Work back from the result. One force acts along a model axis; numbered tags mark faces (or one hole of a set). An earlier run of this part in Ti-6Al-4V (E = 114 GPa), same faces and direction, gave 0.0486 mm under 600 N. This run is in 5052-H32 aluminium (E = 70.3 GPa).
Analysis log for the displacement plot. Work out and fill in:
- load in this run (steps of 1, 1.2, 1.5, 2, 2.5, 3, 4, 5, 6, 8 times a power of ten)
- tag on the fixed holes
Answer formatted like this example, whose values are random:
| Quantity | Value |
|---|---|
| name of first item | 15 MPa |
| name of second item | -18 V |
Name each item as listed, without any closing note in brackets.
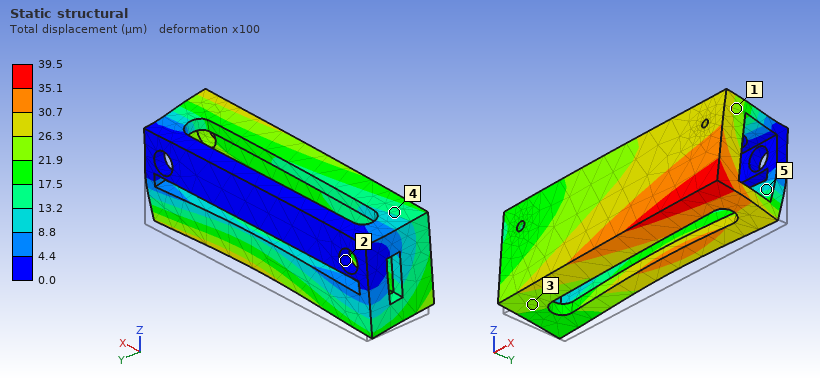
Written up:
| Quantity | Value |
|---|---|
| load in this run | 300 N |
| tag on the fixed holes | 2 |
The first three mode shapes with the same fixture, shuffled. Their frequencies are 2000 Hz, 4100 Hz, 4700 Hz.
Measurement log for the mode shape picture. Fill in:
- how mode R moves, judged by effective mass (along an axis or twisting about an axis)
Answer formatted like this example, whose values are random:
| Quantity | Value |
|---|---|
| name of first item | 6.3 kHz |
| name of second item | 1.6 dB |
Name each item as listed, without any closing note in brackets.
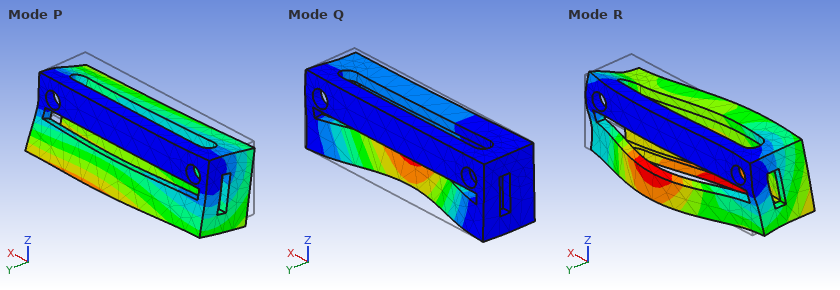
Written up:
| Quantity | Value |
|---|---|
| how mode R moves, judged by effective mass | along X |
